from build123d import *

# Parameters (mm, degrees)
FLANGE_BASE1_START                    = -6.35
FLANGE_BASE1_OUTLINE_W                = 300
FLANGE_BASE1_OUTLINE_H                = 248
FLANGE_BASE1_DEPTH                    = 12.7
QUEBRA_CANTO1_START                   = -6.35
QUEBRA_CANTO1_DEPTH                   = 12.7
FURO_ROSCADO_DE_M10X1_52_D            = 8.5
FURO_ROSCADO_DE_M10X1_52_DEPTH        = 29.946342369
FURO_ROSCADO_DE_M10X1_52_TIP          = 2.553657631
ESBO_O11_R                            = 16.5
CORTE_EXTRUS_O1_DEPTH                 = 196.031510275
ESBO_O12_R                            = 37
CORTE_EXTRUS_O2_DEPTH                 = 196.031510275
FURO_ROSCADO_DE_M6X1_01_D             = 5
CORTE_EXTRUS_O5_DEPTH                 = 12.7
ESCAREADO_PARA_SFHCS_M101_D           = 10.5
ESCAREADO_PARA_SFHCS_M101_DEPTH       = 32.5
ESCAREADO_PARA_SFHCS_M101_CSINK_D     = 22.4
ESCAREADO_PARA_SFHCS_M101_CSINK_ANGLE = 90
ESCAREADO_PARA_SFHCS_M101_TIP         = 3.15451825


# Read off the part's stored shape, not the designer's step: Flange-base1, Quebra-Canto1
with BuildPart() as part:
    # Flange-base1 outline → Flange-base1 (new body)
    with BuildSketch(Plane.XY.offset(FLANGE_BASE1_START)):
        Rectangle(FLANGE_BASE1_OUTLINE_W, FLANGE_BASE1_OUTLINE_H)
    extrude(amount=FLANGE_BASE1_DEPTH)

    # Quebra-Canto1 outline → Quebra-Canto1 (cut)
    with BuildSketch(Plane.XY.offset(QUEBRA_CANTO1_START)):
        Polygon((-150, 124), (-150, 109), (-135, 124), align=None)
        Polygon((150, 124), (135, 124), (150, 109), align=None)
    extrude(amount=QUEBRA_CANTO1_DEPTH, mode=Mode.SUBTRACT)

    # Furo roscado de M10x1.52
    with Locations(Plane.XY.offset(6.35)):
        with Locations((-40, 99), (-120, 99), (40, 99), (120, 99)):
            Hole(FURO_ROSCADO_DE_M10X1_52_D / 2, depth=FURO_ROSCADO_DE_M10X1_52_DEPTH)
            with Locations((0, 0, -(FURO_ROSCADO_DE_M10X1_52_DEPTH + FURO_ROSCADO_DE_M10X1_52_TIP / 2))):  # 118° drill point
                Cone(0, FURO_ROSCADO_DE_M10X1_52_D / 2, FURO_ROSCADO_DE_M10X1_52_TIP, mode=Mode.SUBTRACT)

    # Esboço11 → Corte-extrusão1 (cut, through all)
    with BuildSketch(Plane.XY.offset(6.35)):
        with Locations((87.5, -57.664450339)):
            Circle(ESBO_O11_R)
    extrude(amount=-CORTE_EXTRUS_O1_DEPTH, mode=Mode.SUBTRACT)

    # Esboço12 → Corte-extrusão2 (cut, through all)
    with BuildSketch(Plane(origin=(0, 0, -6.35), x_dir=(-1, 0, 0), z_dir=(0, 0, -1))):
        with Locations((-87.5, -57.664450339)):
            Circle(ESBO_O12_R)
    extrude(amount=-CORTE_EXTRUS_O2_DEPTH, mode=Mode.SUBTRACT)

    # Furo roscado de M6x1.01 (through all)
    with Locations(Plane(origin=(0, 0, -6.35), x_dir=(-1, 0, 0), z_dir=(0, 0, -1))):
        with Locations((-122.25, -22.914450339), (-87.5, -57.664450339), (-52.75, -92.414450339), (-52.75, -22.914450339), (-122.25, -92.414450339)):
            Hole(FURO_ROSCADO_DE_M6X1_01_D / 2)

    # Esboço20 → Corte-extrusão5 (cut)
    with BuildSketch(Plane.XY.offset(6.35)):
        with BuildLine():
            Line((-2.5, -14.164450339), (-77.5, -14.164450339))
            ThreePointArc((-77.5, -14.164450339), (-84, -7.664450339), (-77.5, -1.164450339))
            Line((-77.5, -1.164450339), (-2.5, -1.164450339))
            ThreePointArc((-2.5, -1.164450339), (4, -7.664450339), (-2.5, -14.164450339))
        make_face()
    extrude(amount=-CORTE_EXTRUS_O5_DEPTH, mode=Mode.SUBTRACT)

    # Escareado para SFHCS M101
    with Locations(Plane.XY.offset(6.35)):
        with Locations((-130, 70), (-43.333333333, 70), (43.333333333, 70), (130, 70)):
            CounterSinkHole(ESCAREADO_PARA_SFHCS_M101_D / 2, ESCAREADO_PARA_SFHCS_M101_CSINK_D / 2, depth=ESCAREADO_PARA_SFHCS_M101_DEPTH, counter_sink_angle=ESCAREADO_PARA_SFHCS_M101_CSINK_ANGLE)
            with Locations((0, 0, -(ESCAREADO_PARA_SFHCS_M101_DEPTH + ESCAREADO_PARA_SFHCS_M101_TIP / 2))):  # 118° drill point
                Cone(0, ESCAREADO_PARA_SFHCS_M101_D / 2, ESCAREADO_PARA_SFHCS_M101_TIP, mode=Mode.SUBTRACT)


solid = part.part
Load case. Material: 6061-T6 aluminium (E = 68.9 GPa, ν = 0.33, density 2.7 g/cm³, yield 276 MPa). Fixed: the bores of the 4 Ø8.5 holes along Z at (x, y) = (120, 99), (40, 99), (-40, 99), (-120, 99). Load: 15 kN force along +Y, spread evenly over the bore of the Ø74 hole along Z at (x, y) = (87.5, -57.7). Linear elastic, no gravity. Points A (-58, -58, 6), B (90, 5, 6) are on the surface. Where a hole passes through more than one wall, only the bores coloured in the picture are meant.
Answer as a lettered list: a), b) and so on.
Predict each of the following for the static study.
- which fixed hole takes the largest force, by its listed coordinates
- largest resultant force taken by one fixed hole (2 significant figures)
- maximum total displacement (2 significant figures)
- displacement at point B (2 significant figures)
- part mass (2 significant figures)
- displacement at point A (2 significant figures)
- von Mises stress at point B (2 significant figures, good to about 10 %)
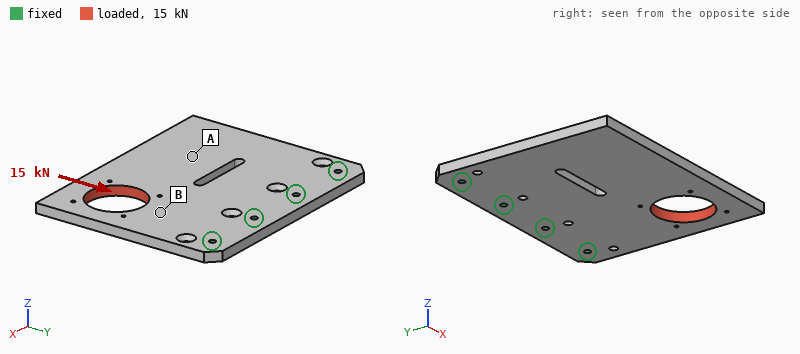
a) (120, 99)
b) 8.9 kN
c) 51 µm
d) 17 µm
e) 2.3 kg
f) 12 µm
g) 6.2 MPa
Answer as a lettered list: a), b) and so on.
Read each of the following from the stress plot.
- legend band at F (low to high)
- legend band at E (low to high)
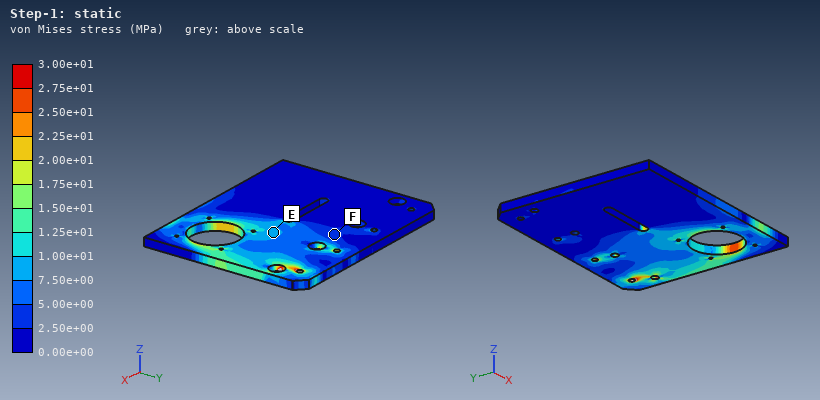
a) 2.50e+00 to 5.00e+00 MPa
b) 7.50e+00 to 1.00e+01 MPa
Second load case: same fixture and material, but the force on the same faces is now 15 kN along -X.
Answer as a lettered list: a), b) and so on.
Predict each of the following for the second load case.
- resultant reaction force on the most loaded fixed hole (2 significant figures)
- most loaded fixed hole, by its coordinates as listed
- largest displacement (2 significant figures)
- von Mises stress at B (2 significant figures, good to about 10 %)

a) 10 kN
b) (120, 99)
c) 86 µm
d) 14 MPa
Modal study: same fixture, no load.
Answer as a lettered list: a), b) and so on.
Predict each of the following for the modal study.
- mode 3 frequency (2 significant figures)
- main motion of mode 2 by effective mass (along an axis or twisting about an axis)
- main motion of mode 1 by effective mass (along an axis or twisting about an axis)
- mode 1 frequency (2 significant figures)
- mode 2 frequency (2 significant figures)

a) 940 Hz
b) twisting about Y
c) along Z
d) 200 Hz
e) 400 Hz
